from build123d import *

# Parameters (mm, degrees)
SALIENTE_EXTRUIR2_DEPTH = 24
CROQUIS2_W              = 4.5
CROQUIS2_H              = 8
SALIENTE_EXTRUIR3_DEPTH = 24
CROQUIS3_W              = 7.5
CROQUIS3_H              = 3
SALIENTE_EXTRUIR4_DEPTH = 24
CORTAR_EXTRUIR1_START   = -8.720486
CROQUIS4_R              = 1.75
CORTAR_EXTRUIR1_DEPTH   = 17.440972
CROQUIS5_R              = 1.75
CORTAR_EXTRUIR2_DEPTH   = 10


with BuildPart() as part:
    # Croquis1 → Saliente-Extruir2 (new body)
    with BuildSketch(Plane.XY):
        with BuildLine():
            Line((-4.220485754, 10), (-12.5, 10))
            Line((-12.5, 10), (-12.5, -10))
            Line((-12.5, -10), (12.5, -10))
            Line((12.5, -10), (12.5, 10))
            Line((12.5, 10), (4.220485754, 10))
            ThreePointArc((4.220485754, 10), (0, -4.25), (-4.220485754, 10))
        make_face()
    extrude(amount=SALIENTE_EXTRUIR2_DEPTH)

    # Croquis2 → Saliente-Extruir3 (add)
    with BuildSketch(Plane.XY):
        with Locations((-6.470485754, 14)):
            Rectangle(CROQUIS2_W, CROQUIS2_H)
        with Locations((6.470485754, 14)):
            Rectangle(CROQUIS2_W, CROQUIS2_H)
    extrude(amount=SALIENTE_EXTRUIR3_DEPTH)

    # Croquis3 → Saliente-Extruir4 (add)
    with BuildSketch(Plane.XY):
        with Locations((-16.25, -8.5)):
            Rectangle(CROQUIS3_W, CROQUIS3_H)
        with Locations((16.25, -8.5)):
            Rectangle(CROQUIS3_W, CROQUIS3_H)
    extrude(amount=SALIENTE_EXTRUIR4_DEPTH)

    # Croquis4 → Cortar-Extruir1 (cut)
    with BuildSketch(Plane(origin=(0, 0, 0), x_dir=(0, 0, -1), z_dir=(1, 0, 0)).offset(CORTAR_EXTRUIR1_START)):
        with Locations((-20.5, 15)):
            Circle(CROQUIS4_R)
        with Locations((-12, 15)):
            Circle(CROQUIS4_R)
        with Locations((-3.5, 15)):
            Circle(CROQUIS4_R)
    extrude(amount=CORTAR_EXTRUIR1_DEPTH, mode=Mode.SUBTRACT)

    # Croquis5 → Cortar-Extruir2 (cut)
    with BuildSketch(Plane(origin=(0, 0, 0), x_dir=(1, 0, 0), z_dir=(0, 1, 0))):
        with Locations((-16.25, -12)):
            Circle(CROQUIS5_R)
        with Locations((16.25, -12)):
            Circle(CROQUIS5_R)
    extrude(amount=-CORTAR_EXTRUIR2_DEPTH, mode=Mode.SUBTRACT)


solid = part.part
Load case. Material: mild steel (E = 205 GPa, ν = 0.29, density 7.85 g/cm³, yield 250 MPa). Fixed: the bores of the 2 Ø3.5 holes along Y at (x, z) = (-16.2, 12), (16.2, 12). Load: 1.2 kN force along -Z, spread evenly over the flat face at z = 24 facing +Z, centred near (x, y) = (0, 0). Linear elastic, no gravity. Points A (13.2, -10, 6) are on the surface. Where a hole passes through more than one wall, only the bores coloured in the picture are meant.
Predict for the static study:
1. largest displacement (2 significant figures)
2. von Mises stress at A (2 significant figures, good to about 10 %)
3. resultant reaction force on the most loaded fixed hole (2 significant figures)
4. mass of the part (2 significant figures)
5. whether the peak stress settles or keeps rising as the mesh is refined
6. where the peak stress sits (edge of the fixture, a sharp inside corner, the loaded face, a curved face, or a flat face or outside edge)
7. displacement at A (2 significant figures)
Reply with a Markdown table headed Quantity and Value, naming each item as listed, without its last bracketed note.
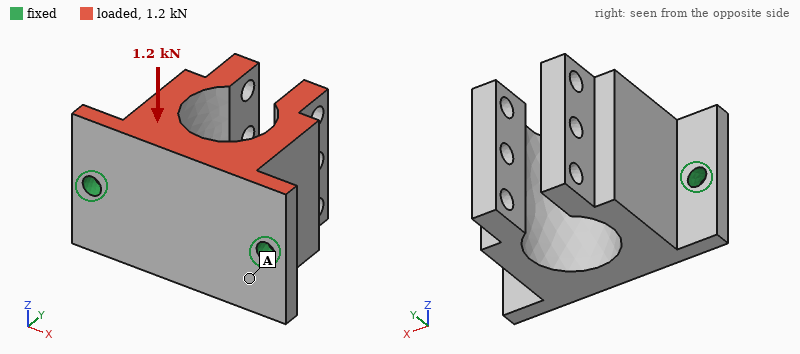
| Quantity | Value |
|---|---|
| largest displacement | 47 µm |
| von Mises stress at A | 31 MPa |
| resultant reaction force on the most loaded fixed hole | 600 N |
| mass of the part | 80 g |
| whether the peak stress settles or keeps rising as the mesh is refined | keeps rising |
| where the peak stress sits | edge of the fixture |
| displacement at A | 8.1 µm |
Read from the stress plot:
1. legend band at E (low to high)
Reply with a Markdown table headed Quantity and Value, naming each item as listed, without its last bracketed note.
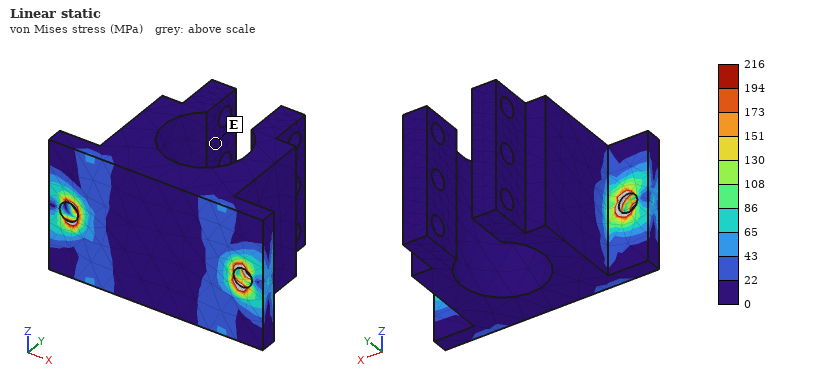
| Quantity | Value |
|---|---|
| legend band at E | 0 to 22 MPa |
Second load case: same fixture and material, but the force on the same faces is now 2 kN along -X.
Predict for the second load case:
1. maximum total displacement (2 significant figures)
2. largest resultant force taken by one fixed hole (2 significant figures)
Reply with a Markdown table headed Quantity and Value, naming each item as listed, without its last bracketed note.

| Quantity | Value |
|---|---|
| maximum total displacement | 29 µm |
| largest resultant force taken by one fixed hole | 1.4 kN |
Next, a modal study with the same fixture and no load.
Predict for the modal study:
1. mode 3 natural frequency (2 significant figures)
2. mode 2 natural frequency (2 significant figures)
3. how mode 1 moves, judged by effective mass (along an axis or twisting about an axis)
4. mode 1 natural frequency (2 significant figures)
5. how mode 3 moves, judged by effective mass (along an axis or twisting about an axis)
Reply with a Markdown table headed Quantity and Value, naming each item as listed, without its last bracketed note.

| Quantity | Value |
|---|---|
| mode 3 natural frequency | 8200 Hz |
| mode 2 natural frequency | 6800 Hz |
| how mode 1 moves, judged by effective mass | along Z |
| mode 1 natural frequency | 3400 Hz |
| how mode 3 moves, judged by effective mass | along X |
